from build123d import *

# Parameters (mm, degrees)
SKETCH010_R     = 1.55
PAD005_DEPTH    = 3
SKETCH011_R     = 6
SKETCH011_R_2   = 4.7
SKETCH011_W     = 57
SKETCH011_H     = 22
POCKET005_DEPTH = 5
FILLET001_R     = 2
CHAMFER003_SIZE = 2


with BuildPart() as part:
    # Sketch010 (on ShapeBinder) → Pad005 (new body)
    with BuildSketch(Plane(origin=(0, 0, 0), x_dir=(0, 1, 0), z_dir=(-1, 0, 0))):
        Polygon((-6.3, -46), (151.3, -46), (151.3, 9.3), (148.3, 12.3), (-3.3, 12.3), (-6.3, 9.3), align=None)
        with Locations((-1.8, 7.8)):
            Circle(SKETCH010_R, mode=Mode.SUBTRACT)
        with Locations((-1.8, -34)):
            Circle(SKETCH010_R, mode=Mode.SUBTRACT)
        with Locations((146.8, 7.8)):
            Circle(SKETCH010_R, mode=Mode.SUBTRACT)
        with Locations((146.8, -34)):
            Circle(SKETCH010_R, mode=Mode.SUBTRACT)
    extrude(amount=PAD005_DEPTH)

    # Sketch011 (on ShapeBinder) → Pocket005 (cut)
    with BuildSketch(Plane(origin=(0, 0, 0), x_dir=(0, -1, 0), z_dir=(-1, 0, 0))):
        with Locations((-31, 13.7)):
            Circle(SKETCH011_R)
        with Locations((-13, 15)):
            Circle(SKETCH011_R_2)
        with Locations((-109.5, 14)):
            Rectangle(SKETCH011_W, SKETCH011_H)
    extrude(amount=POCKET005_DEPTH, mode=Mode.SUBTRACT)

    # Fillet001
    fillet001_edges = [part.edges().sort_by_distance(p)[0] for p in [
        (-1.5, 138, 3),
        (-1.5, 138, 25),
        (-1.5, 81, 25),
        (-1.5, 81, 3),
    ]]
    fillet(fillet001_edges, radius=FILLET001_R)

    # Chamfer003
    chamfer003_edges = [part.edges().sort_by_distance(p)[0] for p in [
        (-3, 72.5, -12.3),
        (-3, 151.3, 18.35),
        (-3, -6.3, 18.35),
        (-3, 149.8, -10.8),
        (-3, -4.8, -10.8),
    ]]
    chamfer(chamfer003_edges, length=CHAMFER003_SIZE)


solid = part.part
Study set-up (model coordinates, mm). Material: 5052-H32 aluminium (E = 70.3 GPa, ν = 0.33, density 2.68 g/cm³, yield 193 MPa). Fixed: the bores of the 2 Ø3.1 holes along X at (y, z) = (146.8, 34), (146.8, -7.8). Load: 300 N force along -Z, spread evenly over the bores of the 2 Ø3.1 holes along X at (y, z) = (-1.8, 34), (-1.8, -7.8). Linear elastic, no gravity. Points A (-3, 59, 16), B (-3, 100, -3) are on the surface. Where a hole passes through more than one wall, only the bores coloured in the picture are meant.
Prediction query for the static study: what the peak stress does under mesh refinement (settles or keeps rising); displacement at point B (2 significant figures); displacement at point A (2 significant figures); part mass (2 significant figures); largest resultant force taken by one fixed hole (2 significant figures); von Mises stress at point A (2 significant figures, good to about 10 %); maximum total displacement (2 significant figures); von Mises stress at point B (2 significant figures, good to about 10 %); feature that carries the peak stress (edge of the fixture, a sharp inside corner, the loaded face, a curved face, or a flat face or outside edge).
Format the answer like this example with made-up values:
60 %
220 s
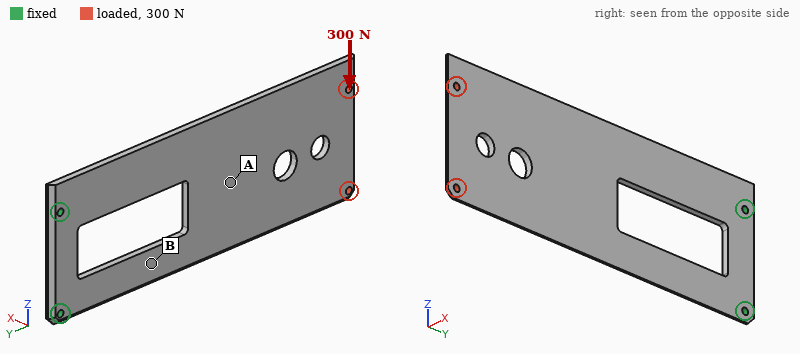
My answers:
keeps rising
0.070 mm
0.13 mm
61 g
1.0 kN
8.1 MPa
0.23 mm
21 MPa
edge of the fixture
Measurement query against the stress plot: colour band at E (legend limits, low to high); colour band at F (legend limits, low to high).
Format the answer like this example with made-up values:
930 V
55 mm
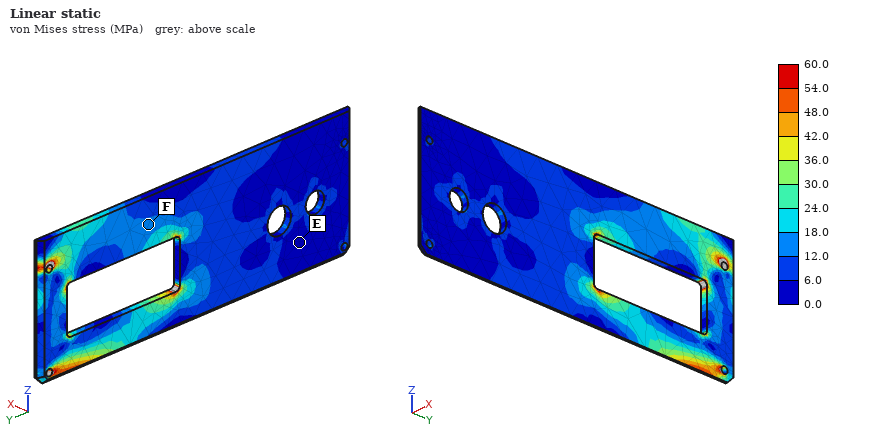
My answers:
0.0 to 6.0 MPa
12.0 to 18.0 MPa
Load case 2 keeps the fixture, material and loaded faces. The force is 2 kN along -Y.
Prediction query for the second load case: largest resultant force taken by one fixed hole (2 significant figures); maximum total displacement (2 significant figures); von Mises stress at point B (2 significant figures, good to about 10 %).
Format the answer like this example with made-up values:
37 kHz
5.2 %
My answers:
1.0 kN
0.10 mm
26 MPa
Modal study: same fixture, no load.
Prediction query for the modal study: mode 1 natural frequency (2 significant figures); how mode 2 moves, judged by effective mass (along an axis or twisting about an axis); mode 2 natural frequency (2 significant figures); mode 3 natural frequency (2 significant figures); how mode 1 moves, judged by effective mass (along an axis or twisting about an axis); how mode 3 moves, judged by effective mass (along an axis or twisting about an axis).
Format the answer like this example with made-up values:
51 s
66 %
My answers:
87 Hz
twisting about Y
490 Hz
630 Hz
along X
along X
